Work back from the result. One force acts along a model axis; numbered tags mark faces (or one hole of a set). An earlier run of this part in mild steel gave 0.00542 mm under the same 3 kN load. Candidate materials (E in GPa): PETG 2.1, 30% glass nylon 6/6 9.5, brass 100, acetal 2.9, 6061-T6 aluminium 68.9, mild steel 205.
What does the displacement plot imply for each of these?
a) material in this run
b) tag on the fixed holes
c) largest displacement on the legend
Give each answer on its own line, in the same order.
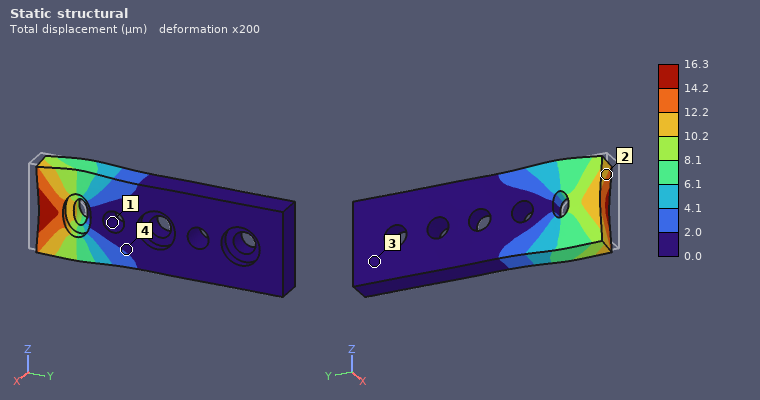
6061-T6 aluminium
1
16.3 µm
